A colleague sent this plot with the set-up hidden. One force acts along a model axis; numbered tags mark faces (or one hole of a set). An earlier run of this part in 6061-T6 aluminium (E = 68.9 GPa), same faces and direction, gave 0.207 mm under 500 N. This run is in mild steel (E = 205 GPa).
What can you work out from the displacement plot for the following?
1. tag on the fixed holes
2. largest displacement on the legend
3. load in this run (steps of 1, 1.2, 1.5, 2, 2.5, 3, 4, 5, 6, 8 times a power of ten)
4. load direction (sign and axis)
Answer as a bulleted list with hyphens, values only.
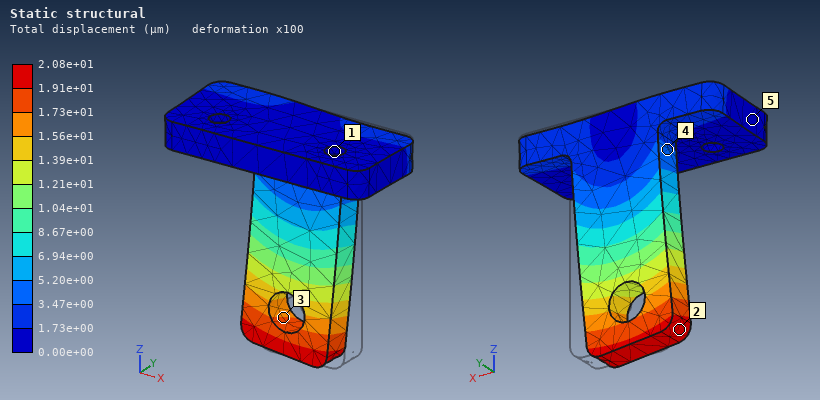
- 1
- 2.08e+01 µm
- 150 N
- -X
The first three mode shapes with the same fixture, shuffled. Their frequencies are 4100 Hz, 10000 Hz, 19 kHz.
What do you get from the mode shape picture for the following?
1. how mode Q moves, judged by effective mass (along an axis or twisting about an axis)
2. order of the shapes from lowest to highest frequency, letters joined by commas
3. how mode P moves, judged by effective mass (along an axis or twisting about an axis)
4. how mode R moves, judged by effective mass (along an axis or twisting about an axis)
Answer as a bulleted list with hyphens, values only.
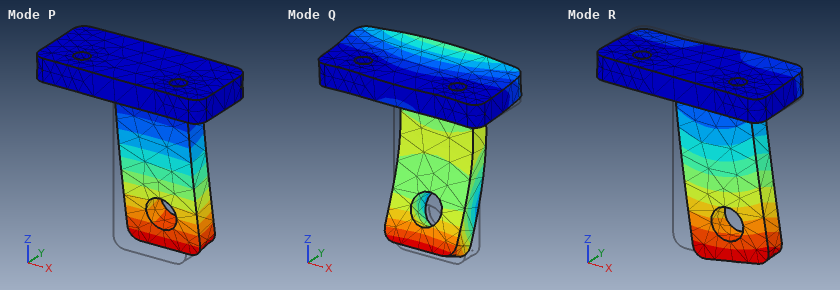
- along Z
- P, R, Q
- along Y
- along X
